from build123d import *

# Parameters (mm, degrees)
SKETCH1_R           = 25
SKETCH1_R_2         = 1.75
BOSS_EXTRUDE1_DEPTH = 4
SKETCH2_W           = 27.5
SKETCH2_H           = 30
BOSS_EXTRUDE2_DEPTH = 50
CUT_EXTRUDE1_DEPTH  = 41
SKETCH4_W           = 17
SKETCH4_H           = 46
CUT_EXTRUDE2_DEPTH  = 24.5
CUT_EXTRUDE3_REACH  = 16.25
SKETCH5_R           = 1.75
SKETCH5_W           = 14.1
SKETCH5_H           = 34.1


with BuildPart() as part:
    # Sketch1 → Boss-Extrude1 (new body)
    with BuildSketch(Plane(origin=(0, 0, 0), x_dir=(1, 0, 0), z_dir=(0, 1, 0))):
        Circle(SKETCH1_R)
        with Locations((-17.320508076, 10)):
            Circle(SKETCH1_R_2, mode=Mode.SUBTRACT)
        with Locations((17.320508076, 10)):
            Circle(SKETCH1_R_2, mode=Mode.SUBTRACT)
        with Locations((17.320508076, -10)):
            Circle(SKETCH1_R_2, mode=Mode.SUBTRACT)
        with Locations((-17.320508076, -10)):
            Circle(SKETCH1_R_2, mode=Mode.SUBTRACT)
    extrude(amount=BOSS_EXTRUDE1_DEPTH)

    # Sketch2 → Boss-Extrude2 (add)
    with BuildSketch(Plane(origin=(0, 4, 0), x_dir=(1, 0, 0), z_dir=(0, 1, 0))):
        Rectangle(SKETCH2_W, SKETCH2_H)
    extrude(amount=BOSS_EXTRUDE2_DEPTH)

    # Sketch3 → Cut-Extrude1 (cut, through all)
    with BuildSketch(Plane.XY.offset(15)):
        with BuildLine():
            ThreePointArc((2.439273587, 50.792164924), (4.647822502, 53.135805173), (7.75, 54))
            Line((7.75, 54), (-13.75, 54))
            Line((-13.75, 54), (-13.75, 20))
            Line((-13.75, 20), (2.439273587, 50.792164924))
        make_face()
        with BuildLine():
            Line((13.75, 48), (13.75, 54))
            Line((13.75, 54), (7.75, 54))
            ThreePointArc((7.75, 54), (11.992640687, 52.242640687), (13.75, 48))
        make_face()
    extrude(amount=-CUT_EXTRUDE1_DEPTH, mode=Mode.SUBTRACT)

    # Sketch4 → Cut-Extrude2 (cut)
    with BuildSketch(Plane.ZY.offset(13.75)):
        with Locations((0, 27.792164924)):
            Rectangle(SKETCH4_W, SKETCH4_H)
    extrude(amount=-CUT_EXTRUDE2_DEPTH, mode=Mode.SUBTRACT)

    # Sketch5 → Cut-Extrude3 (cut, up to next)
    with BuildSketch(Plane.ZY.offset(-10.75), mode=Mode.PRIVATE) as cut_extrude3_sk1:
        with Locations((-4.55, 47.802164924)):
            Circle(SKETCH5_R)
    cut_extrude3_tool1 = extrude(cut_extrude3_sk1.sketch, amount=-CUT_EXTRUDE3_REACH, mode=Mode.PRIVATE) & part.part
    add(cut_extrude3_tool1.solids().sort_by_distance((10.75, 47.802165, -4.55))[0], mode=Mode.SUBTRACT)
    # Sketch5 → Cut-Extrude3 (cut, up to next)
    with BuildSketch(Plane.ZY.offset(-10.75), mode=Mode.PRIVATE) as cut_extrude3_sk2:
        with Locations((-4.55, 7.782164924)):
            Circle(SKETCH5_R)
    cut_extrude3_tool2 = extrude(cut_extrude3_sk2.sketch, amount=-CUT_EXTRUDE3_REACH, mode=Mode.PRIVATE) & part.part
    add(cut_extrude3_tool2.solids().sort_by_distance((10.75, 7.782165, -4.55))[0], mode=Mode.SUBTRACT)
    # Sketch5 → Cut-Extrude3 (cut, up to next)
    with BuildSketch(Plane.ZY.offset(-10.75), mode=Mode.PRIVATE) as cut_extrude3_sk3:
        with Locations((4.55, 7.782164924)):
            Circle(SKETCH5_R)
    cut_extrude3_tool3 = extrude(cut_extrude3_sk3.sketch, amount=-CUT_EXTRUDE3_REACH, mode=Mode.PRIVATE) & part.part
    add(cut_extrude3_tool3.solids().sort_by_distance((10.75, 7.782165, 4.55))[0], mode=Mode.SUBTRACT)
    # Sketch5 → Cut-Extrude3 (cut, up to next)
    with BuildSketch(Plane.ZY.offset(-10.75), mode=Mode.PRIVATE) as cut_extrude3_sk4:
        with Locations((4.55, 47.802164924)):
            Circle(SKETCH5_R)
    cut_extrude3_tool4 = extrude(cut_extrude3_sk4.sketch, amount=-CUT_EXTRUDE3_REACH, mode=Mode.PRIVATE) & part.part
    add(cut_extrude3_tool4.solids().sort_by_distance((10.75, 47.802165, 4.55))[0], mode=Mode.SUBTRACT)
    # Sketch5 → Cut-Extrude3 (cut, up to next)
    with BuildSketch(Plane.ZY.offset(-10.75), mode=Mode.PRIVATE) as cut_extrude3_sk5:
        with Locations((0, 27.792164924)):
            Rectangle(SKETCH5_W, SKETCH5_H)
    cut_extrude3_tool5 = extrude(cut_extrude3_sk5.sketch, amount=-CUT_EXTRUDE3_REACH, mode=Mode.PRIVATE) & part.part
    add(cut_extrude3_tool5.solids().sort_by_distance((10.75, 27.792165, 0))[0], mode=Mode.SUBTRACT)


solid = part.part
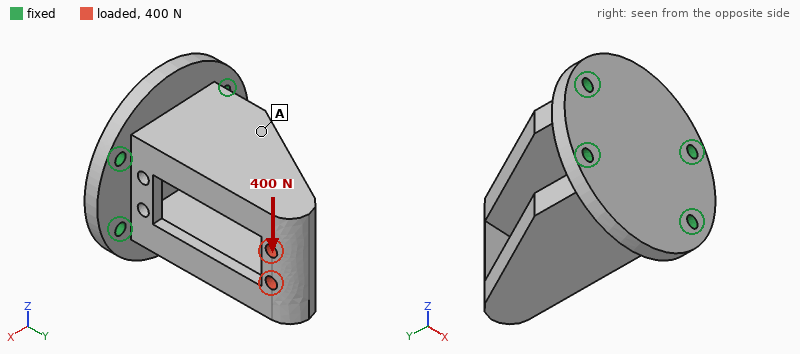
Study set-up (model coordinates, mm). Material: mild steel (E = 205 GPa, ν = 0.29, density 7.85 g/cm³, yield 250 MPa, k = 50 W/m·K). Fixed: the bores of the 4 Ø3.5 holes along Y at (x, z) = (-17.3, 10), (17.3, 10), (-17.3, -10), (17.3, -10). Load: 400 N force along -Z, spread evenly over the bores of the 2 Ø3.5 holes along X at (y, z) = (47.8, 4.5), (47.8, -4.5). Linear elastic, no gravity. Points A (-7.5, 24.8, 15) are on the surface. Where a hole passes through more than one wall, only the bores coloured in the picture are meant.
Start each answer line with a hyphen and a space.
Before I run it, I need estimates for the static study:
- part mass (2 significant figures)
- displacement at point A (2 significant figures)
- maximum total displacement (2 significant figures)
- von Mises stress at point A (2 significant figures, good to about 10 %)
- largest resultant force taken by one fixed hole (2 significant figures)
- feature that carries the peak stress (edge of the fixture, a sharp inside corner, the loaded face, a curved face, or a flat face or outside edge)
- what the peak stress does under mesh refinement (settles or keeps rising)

- 180 g
- 13 µm
- 38 µm
- 12 MPa
- 470 N
- a sharp inside corner
- keeps rising
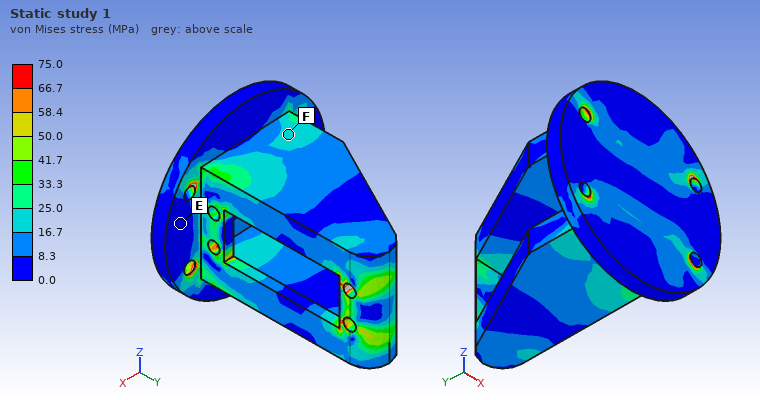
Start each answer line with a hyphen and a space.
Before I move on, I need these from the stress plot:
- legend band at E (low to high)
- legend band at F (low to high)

- 0.0 to 8.3 MPa
- 16.7 to 25.0 MPa
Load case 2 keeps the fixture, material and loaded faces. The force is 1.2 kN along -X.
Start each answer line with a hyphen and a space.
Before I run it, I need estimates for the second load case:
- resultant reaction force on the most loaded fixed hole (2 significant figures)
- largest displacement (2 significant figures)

- 970 N
- 29 µm
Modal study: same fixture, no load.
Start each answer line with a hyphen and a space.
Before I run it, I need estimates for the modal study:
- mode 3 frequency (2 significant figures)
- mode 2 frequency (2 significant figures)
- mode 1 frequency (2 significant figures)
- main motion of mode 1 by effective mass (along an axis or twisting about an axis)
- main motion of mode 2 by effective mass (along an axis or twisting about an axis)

- 8100 Hz
- 6600 Hz
- 2800 Hz
- along Z
- along X
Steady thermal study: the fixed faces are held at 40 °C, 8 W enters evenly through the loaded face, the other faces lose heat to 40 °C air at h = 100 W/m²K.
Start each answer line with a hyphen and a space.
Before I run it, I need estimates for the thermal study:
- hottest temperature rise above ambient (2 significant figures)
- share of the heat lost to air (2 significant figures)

- 34 K
- 69 %
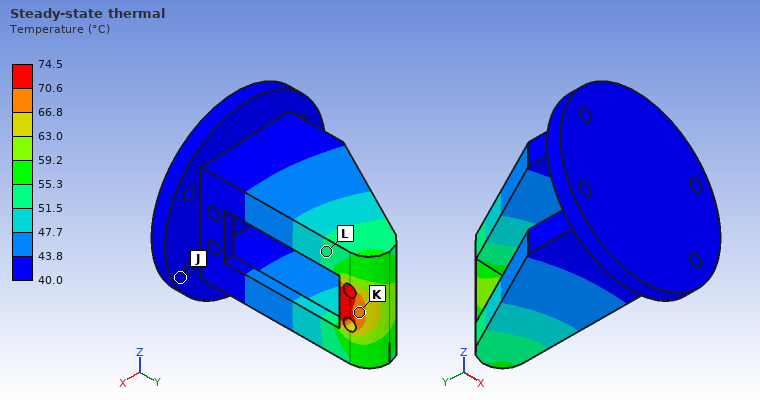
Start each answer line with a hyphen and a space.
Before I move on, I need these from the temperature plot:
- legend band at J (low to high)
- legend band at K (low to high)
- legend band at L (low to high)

- 40.0 to 43.8 °C
- 66.8 to 70.6 °C
- 51.5 to 55.3 °C
